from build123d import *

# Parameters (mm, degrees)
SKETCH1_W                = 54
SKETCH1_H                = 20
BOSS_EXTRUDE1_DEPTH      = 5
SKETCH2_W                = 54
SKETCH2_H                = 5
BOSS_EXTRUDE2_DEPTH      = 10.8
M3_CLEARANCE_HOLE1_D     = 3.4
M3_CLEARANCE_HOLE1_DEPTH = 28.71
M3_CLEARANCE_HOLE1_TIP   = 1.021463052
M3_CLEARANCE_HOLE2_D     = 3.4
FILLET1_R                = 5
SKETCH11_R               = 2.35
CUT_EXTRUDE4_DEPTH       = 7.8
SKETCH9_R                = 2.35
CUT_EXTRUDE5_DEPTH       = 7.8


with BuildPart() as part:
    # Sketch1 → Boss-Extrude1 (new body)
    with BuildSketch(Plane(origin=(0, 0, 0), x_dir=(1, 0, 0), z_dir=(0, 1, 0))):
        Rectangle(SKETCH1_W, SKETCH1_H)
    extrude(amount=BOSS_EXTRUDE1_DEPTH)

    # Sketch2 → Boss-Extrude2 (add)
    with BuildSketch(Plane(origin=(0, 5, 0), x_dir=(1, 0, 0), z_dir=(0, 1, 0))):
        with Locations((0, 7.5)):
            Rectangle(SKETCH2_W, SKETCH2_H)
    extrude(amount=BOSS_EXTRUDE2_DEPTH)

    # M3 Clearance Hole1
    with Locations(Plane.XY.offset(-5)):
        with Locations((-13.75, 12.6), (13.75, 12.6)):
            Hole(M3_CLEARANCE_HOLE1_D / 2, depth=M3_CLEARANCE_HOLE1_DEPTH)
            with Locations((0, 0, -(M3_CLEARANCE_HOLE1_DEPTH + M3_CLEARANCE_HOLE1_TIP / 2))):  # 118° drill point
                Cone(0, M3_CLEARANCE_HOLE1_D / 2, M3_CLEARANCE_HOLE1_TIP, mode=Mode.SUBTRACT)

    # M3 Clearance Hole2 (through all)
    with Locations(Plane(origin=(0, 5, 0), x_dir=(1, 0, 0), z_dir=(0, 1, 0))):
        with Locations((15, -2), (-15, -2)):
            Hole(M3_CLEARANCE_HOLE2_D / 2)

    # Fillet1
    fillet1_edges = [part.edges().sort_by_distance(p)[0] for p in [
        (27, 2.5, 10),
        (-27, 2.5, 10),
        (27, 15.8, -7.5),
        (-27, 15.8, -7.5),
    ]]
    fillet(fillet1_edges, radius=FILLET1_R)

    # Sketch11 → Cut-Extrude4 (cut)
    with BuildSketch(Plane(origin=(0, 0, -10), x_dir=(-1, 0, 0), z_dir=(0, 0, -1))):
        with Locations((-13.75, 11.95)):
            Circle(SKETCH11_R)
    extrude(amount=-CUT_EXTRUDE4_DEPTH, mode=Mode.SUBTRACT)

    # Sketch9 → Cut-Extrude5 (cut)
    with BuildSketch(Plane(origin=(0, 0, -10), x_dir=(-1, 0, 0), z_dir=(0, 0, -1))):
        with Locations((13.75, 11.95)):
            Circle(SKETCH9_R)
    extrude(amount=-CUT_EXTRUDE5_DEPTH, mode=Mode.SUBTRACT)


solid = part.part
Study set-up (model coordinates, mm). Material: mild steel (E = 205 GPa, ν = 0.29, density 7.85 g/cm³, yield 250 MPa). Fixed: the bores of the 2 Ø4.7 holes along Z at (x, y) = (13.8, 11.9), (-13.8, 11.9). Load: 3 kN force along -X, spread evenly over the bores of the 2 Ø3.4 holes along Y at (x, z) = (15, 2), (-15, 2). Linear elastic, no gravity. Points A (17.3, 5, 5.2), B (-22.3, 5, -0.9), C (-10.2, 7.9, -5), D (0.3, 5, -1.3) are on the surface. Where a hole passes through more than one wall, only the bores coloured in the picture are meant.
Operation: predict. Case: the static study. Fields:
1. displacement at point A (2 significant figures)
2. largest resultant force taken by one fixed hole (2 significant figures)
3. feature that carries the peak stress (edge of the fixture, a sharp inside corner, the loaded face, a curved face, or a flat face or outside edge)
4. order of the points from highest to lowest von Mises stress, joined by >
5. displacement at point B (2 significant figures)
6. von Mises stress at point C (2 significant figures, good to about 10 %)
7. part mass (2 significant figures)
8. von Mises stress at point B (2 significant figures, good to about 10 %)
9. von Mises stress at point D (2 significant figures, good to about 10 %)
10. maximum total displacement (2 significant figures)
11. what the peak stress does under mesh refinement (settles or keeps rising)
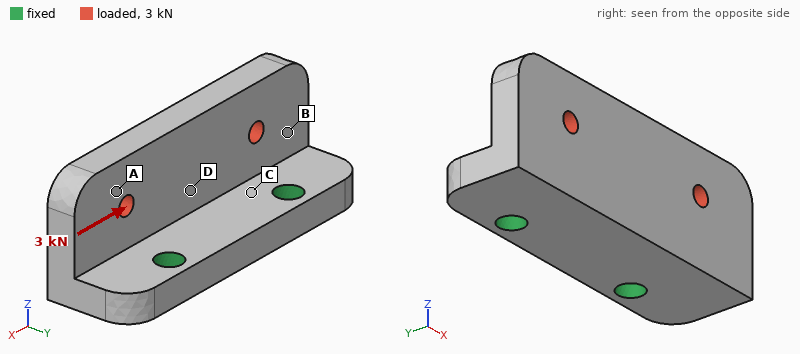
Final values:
10.0 µm
1.9 kN
edge of the fixture
C > D > B > A
8.1 µm
59 MPa
62 g
23 MPa
41 MPa
14 µm
keeps rising
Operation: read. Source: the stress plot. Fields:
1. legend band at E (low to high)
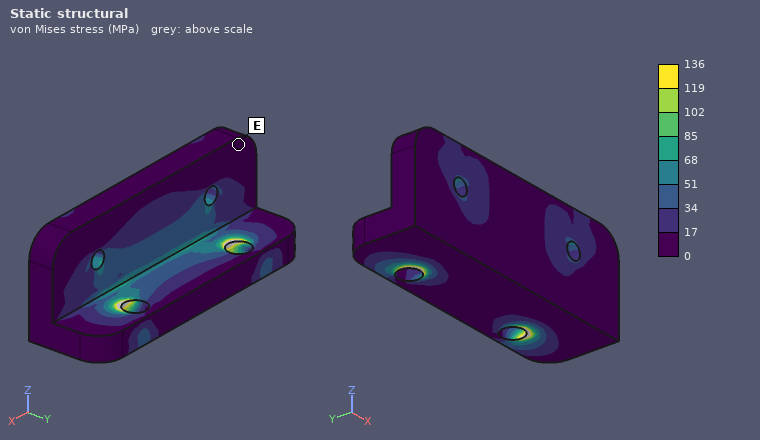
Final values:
0 to 17 MPa
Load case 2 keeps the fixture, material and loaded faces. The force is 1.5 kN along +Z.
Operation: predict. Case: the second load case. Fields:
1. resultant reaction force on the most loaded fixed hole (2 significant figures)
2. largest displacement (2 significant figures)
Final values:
750 N
15 µm
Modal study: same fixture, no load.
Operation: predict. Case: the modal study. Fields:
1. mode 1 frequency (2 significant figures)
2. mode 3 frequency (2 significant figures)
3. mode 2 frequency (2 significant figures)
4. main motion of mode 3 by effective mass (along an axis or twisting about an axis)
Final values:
6900 Hz
16 kHz
9800 Hz
along X
